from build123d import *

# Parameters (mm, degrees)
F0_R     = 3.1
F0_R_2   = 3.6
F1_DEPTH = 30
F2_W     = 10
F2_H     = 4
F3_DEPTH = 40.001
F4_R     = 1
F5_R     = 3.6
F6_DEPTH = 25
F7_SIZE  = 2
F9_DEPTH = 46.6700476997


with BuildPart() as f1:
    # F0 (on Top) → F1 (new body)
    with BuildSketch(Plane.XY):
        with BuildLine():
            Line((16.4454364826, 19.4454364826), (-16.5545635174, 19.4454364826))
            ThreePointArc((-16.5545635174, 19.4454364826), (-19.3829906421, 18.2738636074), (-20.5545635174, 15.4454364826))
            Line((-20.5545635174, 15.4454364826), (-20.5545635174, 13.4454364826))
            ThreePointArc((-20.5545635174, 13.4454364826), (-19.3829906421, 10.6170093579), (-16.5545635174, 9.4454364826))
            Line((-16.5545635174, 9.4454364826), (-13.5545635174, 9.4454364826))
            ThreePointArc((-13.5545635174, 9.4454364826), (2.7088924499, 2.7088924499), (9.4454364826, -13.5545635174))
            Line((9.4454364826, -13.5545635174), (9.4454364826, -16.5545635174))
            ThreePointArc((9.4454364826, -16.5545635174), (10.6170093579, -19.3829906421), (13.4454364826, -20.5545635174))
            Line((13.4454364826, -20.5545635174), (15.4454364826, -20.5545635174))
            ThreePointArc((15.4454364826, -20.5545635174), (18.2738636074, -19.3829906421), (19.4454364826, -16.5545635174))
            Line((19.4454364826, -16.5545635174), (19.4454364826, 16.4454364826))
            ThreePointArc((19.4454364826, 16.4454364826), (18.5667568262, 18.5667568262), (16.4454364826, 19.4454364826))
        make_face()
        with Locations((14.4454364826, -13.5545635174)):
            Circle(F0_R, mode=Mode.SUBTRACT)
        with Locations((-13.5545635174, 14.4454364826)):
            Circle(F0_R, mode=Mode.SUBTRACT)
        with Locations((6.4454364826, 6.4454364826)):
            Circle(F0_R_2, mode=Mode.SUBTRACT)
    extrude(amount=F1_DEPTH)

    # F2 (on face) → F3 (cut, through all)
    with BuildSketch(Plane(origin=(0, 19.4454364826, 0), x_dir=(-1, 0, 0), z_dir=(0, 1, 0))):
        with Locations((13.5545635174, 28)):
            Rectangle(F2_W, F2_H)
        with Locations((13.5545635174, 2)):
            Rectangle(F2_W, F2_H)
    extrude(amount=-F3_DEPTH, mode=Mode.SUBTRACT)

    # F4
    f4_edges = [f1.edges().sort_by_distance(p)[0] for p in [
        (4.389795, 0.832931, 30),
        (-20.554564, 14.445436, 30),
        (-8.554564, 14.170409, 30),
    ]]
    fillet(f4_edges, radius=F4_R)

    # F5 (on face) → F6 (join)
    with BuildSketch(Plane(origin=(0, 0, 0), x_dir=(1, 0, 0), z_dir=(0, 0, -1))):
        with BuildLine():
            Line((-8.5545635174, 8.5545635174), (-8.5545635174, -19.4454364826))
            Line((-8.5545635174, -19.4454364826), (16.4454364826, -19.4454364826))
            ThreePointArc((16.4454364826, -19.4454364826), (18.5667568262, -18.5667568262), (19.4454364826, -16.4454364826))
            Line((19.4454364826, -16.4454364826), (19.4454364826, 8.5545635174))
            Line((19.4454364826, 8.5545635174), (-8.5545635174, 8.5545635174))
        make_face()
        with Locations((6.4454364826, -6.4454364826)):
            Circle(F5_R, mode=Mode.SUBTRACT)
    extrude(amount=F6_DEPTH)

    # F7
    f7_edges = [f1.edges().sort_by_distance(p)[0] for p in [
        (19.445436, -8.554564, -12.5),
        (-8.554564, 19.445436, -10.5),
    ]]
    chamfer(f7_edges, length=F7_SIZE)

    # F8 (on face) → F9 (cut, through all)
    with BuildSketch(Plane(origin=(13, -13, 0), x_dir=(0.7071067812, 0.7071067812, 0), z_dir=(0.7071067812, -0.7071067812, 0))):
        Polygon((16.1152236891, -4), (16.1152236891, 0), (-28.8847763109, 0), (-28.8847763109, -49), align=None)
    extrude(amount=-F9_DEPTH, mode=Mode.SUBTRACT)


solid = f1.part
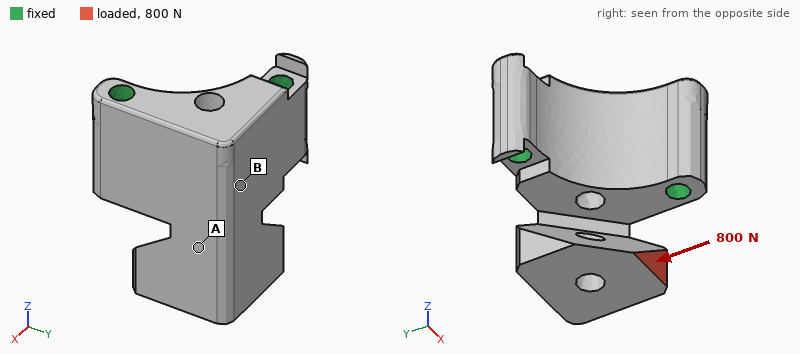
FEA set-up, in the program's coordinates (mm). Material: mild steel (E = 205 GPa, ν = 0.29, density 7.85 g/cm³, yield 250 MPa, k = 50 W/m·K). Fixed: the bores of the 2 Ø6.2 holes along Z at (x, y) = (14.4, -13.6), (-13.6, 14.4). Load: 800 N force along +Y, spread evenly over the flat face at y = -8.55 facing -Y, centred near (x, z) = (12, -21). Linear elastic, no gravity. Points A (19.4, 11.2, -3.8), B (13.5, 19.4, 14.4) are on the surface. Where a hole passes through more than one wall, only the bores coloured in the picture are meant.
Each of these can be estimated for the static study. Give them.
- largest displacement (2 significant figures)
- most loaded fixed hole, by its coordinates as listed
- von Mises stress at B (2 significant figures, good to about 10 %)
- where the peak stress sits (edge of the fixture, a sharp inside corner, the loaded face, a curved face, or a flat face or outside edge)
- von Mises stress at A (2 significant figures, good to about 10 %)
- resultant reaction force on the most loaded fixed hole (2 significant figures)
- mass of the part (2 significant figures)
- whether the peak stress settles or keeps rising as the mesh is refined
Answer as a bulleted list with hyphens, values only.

- 39 µm
- (14.4, -13.6)
- 14 MPa
- a sharp inside corner
- 30 MPa
- 830 N
- 230 g
- keeps rising
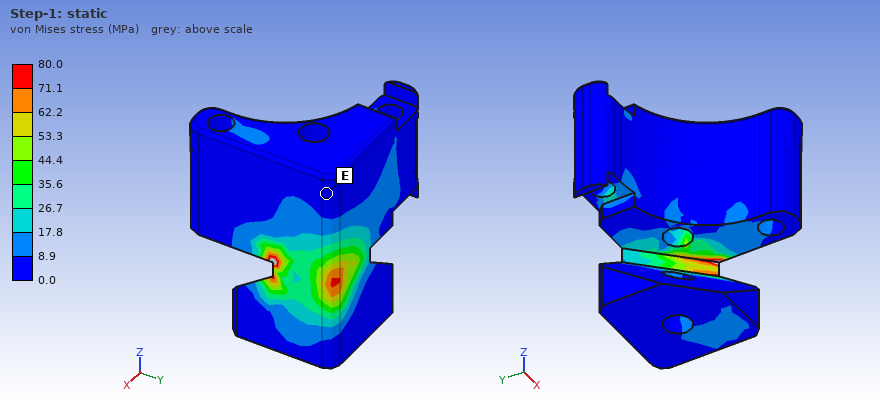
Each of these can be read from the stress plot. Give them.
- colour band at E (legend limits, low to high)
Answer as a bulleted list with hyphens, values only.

- 0.0 to 8.9 MPa
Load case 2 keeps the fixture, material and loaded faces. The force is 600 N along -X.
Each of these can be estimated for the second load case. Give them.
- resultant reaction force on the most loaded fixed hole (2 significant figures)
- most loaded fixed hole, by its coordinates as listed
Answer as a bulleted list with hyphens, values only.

- 610 N
- (14.4, -13.6)
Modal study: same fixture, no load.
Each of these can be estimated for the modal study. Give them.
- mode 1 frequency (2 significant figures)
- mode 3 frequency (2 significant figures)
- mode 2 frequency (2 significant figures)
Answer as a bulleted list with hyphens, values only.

- 3300 Hz
- 8200 Hz
- 4300 Hz
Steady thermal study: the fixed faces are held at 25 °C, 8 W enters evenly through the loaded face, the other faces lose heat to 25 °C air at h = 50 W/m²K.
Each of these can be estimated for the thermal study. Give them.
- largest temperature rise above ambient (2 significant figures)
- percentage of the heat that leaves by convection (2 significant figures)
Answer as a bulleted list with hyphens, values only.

- 34 K
- 41 %
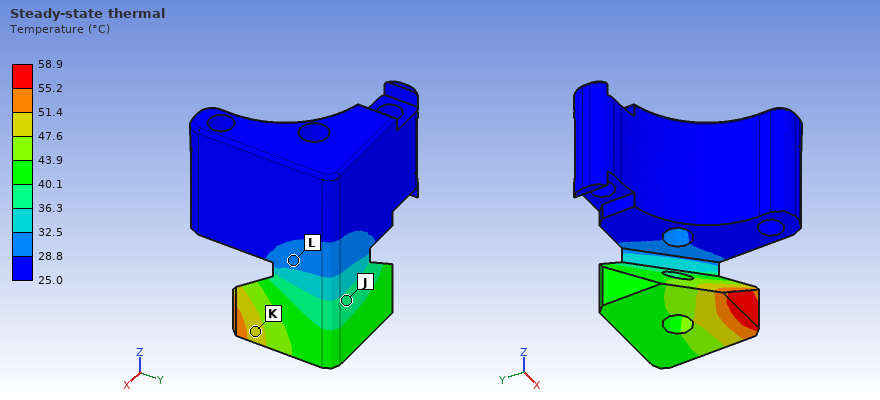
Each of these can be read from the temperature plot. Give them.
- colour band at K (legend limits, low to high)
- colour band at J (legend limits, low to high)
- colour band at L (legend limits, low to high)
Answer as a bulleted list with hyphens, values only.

- 47.6 to 51.4 °C
- 36.3 to 40.1 °C
- 28.8 to 32.5 °C
